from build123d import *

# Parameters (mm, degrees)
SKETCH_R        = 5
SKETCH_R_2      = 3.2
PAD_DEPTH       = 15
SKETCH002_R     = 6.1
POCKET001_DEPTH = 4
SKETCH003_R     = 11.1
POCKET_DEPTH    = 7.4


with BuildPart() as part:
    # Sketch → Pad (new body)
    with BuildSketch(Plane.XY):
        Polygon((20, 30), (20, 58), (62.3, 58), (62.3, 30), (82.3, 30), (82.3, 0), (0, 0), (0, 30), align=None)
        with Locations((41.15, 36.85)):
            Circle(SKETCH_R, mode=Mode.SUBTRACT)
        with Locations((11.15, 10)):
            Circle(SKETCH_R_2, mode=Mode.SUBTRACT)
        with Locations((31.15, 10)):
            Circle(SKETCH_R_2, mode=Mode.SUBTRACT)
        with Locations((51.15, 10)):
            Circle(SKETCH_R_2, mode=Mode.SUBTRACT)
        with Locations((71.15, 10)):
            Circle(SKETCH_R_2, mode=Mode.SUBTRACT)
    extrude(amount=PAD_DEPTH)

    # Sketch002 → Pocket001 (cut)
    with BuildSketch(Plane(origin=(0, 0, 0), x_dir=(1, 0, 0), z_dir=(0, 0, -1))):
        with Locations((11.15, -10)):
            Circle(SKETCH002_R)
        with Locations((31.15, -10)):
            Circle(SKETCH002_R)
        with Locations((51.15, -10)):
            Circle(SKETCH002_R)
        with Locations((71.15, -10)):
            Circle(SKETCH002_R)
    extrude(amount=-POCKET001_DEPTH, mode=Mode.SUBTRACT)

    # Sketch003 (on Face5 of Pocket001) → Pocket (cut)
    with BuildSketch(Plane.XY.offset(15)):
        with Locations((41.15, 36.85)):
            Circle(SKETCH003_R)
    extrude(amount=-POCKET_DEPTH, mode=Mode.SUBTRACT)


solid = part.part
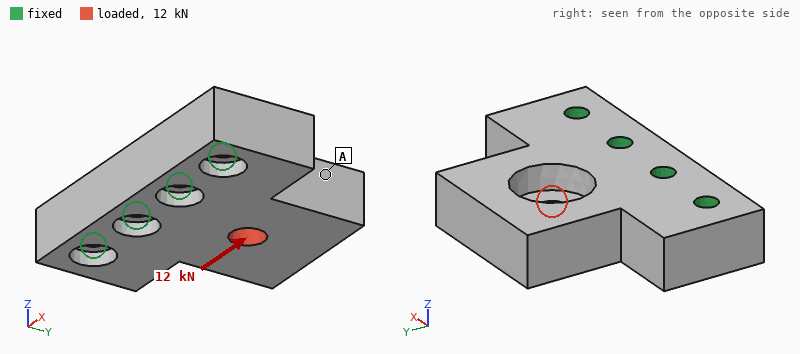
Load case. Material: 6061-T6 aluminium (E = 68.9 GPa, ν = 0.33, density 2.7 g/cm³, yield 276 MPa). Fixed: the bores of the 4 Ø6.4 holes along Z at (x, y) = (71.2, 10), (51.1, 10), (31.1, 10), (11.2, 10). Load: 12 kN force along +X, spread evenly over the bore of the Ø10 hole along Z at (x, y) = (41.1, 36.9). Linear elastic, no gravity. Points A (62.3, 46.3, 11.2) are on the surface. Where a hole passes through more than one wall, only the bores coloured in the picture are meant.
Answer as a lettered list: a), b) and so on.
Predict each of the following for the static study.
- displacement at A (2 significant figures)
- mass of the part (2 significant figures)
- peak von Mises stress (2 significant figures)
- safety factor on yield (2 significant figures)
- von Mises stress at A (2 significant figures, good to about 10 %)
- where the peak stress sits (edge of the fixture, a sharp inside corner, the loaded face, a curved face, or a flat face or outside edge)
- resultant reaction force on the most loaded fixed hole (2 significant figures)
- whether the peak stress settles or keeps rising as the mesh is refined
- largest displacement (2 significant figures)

a) 28 µm
b) 130 g
c) 120 MPa
d) 2.4
e) 13 MPa
f) the loaded face
g) 5.5 kN
h) settles
i) 37 µm
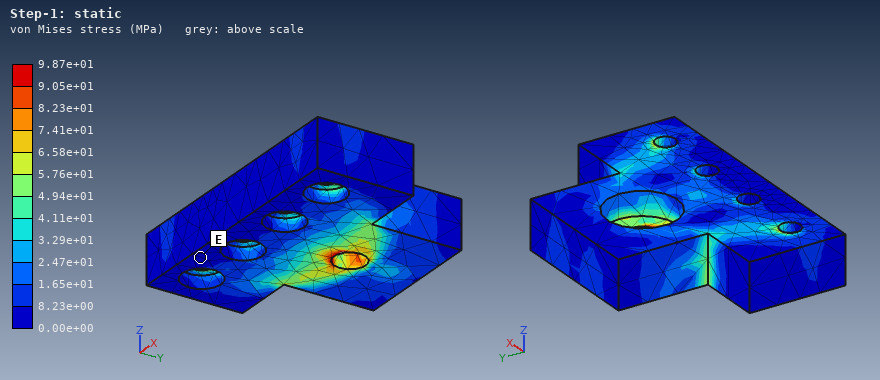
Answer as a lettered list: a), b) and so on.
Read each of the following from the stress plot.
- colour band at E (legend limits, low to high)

a) 0.00e+00 to 8.23e+00 MPa
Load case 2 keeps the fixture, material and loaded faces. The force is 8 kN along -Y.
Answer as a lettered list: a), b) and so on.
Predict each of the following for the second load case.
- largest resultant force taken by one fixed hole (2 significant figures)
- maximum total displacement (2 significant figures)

a) 2.9 kN
b) 42 µm
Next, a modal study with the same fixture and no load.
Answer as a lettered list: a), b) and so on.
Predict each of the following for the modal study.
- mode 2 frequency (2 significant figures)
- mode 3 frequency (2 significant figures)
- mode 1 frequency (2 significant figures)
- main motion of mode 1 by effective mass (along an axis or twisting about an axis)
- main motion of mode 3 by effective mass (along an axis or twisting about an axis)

a) 10 kHz
b) 13 kHz
c) 4900 Hz
d) along Z
e) along X
